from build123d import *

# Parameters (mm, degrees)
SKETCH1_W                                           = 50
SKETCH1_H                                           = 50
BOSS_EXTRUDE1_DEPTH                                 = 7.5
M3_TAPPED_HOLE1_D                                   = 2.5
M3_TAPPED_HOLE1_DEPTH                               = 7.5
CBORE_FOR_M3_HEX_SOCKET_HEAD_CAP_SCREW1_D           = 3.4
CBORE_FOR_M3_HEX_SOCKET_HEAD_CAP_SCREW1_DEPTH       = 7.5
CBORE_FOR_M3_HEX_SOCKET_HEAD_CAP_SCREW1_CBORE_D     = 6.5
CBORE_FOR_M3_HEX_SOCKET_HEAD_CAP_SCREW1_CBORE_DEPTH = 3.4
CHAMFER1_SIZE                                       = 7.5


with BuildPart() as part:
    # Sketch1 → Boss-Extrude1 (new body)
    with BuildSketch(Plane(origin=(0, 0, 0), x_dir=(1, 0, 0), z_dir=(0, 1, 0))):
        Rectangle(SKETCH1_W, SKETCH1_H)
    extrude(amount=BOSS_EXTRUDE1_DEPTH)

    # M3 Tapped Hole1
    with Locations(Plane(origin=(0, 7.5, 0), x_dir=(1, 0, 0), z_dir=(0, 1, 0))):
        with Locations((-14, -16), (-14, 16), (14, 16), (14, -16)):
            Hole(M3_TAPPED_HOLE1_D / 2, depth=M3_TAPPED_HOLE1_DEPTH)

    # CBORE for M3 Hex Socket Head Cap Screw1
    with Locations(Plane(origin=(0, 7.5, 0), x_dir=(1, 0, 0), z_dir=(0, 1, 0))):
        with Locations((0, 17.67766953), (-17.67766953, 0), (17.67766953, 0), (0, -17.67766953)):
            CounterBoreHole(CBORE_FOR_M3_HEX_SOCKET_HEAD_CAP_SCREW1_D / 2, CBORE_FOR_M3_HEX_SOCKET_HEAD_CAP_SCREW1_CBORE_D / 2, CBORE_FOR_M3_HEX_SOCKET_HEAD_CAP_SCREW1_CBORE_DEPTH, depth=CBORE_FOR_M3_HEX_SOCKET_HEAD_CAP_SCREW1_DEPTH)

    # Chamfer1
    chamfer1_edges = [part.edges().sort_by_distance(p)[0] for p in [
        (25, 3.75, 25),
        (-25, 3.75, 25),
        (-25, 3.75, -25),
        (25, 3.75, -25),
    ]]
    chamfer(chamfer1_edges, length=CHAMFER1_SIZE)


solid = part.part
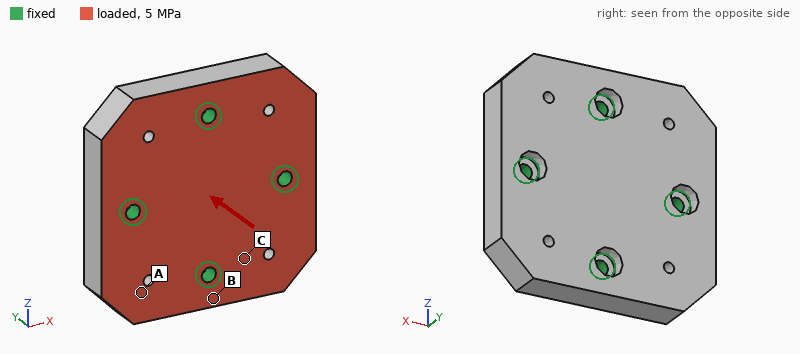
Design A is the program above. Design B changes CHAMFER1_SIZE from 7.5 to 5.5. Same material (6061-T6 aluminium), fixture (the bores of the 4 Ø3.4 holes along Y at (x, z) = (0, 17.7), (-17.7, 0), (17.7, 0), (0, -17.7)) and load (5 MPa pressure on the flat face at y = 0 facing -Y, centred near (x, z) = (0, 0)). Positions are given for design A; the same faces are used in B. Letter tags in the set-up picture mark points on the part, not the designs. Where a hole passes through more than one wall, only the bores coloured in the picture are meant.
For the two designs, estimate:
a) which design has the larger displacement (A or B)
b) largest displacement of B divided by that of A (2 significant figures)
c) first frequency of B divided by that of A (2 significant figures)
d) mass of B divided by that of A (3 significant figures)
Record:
B
1.2
0.94
1.02
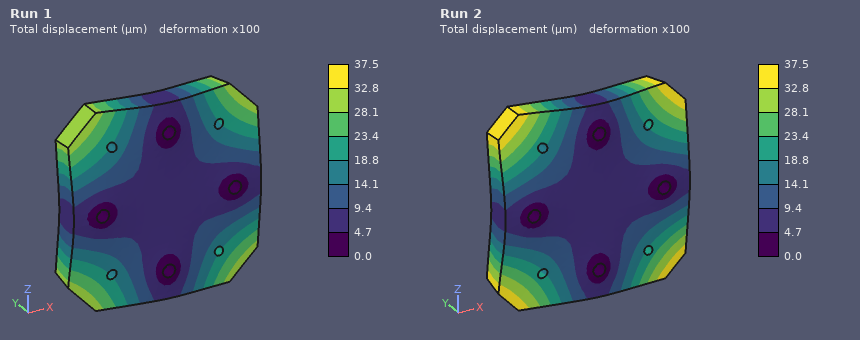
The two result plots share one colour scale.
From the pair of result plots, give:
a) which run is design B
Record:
Run 2
